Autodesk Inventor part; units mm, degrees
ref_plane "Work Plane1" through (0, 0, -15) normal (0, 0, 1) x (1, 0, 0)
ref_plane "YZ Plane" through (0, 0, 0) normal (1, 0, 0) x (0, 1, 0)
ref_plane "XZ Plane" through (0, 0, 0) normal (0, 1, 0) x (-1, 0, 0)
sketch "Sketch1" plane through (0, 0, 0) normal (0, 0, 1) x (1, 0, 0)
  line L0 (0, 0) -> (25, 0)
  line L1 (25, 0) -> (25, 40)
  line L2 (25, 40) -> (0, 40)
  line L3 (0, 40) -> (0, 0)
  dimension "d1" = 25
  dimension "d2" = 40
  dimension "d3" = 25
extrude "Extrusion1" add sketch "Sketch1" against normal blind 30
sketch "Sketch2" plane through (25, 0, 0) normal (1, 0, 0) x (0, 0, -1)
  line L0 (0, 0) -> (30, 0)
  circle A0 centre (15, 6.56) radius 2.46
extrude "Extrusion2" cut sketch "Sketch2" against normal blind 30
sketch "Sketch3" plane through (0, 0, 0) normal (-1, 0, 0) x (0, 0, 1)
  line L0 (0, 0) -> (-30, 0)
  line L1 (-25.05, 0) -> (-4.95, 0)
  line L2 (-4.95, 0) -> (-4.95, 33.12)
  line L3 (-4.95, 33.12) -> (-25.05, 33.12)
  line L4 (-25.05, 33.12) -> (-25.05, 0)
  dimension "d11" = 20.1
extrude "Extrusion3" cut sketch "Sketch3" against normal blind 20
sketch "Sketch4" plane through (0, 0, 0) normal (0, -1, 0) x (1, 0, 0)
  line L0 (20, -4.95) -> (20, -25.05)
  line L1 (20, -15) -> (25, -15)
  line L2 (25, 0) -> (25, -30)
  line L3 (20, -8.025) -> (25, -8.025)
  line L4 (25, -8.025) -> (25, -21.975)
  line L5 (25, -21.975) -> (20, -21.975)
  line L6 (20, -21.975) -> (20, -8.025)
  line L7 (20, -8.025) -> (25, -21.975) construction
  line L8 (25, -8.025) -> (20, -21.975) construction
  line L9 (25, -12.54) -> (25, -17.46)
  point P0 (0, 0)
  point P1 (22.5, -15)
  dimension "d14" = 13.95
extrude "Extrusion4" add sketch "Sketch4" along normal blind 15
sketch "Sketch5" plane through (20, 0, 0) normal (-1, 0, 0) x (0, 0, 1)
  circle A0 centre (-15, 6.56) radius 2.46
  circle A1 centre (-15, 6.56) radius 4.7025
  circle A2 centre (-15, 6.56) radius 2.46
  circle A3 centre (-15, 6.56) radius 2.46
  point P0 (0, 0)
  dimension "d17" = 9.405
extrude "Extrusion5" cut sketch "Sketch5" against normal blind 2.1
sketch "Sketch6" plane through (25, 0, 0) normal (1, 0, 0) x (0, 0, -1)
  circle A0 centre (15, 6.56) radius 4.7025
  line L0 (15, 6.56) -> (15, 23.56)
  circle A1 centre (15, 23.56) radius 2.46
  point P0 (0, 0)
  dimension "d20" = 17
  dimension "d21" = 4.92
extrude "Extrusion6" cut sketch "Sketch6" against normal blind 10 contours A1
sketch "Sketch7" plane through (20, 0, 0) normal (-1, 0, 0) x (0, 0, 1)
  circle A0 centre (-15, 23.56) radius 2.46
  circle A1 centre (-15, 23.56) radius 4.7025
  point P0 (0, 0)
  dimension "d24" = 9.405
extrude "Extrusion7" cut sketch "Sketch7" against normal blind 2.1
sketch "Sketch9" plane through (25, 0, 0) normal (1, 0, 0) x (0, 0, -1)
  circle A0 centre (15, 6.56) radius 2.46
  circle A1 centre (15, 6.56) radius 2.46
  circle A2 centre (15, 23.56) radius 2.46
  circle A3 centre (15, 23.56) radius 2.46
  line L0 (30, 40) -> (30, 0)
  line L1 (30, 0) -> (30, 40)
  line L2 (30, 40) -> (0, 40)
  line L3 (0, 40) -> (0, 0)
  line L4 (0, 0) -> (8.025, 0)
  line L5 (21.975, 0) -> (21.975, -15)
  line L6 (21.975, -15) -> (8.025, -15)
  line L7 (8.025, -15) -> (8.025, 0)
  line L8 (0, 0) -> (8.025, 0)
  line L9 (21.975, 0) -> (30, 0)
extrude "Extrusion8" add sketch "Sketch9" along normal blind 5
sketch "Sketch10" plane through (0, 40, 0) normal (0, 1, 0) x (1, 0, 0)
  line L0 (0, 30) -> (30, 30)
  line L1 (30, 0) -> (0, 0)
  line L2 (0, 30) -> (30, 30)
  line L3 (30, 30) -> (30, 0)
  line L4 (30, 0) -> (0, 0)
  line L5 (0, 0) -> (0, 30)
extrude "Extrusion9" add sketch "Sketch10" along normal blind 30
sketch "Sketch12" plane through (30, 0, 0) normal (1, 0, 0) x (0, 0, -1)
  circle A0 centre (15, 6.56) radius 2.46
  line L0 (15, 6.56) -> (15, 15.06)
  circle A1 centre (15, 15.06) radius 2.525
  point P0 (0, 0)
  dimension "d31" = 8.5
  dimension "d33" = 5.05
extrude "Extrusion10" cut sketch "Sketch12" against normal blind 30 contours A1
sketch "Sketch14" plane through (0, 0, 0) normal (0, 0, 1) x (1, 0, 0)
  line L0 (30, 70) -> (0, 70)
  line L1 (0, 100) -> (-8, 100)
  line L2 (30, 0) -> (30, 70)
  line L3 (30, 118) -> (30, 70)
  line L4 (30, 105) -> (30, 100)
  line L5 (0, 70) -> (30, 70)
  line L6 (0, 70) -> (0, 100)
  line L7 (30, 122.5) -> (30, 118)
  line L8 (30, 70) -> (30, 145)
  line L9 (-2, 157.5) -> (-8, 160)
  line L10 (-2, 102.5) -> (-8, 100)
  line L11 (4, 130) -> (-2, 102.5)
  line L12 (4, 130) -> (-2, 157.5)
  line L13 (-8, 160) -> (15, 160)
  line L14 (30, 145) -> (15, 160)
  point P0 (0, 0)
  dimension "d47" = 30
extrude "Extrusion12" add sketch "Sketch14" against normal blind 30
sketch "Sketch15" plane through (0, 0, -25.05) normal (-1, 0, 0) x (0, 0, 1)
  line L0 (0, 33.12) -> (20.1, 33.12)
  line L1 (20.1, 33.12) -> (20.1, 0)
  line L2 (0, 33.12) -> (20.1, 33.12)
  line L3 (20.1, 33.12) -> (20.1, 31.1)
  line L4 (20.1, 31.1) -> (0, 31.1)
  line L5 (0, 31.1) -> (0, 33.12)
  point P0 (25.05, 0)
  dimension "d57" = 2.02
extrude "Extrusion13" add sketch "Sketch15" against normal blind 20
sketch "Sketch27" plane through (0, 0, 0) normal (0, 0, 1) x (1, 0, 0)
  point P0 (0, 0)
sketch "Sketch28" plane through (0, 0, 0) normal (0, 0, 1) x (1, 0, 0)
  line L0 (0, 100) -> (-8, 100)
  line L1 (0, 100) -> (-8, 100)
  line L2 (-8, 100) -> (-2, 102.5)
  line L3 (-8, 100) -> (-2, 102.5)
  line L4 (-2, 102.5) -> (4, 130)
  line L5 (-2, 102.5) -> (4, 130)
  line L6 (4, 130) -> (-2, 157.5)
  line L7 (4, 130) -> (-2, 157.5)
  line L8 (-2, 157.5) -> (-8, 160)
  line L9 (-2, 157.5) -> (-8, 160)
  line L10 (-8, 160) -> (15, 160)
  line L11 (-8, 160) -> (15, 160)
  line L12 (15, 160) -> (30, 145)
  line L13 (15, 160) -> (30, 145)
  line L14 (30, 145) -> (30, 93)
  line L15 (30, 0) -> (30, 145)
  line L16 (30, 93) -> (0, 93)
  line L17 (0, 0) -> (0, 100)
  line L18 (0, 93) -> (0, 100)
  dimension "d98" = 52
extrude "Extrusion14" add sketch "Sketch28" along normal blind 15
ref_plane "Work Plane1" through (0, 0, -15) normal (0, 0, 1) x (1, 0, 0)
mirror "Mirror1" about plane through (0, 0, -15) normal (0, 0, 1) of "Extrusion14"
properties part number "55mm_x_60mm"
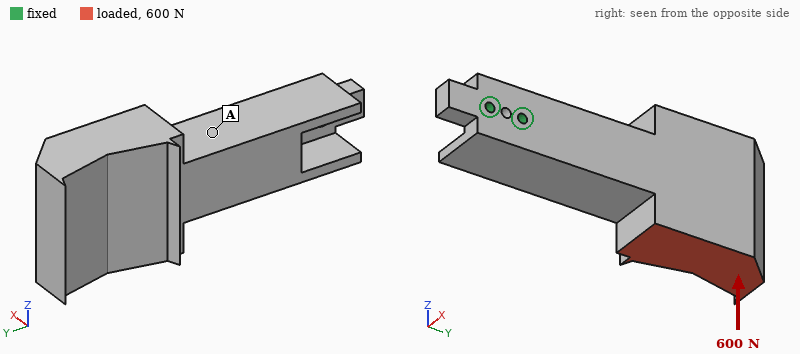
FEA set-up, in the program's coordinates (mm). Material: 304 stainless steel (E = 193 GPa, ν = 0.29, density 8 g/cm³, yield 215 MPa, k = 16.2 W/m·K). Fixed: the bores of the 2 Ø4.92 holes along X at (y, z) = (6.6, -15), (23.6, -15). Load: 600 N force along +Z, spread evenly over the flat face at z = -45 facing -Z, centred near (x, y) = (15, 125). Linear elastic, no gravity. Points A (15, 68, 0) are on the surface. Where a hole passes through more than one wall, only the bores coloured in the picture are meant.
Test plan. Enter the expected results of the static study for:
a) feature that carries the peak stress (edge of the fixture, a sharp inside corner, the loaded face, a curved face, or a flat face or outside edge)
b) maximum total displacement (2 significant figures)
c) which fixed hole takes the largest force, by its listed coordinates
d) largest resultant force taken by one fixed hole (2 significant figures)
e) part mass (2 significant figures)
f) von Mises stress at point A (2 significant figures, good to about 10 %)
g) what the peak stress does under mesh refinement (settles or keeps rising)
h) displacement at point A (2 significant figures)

edge of the fixture
66 µm
(23.6, -15)
3.2 kN
1.5 kg
7.6 MPa
keeps rising
18 µm
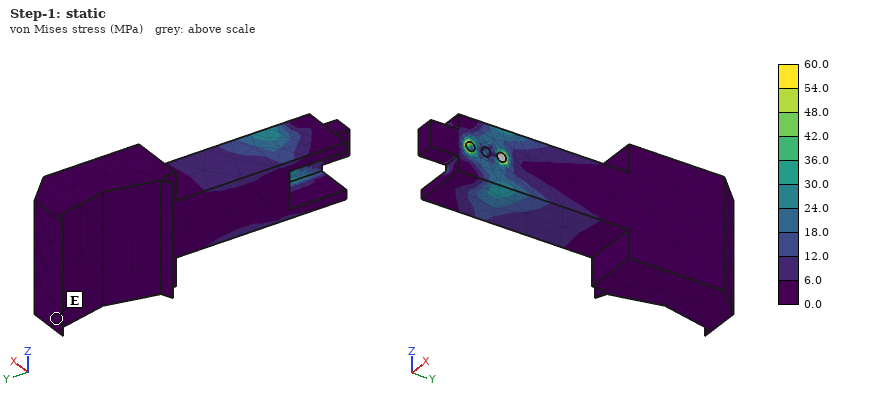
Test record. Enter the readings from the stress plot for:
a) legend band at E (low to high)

0.0 to 6.0 MPa
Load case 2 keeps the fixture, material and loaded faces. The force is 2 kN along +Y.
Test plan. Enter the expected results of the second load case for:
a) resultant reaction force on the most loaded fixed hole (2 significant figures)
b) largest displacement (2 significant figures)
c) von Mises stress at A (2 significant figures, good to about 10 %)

3.0 kN
84 µm
11 MPa
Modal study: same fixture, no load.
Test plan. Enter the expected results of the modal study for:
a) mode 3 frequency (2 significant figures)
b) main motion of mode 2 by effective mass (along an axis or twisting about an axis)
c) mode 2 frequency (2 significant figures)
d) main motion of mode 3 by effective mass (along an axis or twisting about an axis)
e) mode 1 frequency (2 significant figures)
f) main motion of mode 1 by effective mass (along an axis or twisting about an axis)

1600 Hz
along Z
560 Hz
twisting about Y
490 Hz
along X
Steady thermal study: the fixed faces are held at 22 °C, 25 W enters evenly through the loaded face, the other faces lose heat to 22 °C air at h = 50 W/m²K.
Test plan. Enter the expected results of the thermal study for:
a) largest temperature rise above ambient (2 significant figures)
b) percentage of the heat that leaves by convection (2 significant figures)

46 K
93 %
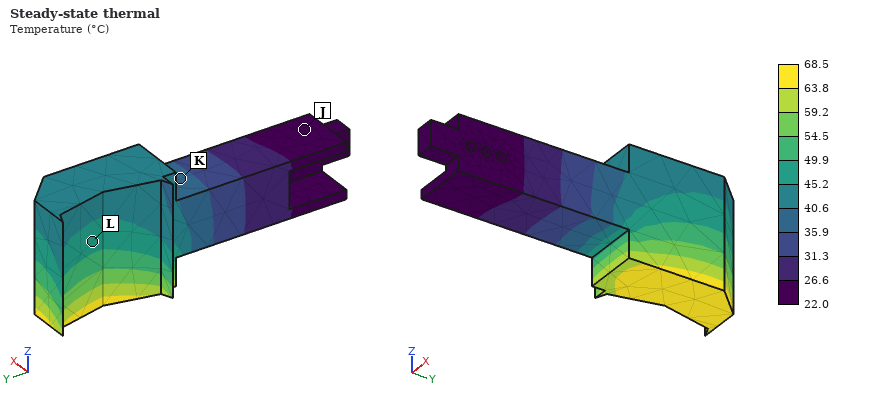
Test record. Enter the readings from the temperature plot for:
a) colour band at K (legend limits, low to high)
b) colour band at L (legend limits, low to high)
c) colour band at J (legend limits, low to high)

35.9 to 40.6 °C
45.2 to 49.9 °C
22.0 to 26.6 °C
